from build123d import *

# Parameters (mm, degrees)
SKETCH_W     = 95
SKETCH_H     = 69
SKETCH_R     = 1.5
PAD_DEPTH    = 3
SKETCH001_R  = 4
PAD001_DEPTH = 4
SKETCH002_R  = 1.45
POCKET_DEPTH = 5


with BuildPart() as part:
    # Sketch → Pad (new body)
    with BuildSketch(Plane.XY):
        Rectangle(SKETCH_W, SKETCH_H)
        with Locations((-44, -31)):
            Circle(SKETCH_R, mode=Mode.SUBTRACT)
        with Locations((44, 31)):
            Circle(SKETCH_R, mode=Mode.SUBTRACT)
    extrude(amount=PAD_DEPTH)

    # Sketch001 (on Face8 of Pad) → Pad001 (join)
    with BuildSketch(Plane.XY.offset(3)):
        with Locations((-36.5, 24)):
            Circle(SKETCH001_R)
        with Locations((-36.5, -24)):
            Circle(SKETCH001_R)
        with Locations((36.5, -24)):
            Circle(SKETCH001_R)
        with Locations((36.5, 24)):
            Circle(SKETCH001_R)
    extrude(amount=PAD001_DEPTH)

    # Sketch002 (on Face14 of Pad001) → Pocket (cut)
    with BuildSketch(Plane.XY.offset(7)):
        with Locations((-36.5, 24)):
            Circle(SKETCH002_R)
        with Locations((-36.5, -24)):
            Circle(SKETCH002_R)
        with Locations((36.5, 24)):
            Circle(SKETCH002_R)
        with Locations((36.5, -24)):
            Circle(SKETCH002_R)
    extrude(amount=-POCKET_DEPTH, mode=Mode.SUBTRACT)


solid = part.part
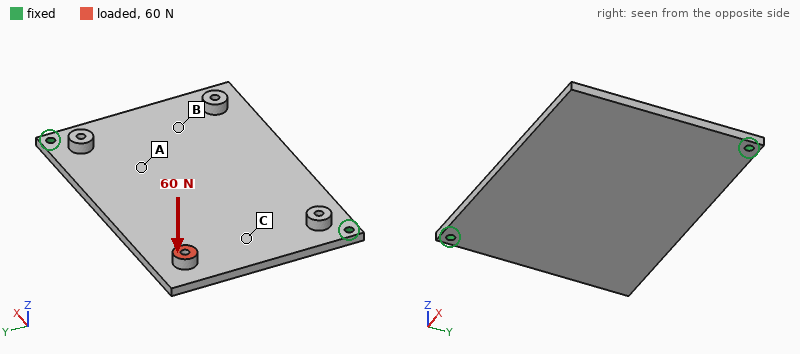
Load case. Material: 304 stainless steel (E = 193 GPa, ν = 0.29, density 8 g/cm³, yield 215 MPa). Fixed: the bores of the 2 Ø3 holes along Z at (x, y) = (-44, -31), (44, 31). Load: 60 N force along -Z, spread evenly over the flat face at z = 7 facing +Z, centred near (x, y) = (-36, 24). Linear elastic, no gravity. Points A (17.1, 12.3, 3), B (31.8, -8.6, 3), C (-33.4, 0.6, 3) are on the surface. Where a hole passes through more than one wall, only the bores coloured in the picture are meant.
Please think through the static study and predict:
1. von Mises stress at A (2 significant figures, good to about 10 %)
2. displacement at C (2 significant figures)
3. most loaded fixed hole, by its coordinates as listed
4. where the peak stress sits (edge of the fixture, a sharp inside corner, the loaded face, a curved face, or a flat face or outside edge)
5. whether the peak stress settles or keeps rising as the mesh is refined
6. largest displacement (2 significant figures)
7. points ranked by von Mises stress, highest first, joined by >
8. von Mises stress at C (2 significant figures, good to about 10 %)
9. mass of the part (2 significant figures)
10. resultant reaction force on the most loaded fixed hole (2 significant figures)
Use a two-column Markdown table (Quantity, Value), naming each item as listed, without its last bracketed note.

| Quantity | Value |
|---|---|
| von Mises stress at A | 12 MPa |
| displacement at C | 0.060 mm |
| most loaded fixed hole, by its coordinates as listed | (-44, -31) |
| where the peak stress sits | edge of the fixture |
| whether the peak stress settles or keeps rising as the mesh is refined | keeps rising |
| largest displacement | 0.19 mm |
| points ranked by von Mises stress, highest first, joined by > | C > A > B |
| von Mises stress at C | 18 MPa |
| mass of the part | 160 g |
| resultant reaction force on the most loaded fixed hole | 41 N |
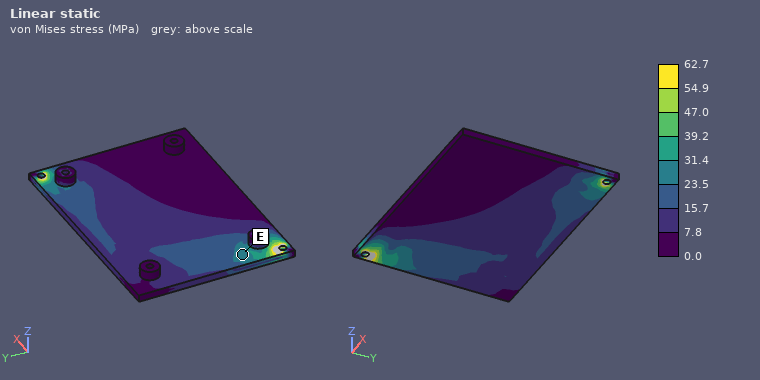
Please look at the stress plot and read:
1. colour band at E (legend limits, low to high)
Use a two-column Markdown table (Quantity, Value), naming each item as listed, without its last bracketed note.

| Quantity | Value |
|---|---|
| colour band at E | 23.5 to 31.4 MPa |
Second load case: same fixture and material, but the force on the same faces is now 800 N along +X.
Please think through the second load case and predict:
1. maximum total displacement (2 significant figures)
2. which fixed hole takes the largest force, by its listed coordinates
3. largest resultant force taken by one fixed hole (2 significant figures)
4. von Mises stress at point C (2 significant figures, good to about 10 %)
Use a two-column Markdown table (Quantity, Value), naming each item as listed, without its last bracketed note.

| Quantity | Value |
|---|---|
| maximum total displacement | 0.23 mm |
| which fixed hole takes the largest force, by its listed coordinates | (44, 31) |
| largest resultant force taken by one fixed hole | 510 N |
| von Mises stress at point C | 47 MPa |
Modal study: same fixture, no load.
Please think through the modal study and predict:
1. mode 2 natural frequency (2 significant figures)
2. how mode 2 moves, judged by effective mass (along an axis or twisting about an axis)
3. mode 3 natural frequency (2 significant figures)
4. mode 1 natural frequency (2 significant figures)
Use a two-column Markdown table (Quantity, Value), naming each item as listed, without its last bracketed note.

| Quantity | Value |
|---|---|
| mode 2 natural frequency | 750 Hz |
| how mode 2 moves, judged by effective mass | along Z |
| mode 3 natural frequency | 1900 Hz |
| mode 1 natural frequency | 580 Hz |
